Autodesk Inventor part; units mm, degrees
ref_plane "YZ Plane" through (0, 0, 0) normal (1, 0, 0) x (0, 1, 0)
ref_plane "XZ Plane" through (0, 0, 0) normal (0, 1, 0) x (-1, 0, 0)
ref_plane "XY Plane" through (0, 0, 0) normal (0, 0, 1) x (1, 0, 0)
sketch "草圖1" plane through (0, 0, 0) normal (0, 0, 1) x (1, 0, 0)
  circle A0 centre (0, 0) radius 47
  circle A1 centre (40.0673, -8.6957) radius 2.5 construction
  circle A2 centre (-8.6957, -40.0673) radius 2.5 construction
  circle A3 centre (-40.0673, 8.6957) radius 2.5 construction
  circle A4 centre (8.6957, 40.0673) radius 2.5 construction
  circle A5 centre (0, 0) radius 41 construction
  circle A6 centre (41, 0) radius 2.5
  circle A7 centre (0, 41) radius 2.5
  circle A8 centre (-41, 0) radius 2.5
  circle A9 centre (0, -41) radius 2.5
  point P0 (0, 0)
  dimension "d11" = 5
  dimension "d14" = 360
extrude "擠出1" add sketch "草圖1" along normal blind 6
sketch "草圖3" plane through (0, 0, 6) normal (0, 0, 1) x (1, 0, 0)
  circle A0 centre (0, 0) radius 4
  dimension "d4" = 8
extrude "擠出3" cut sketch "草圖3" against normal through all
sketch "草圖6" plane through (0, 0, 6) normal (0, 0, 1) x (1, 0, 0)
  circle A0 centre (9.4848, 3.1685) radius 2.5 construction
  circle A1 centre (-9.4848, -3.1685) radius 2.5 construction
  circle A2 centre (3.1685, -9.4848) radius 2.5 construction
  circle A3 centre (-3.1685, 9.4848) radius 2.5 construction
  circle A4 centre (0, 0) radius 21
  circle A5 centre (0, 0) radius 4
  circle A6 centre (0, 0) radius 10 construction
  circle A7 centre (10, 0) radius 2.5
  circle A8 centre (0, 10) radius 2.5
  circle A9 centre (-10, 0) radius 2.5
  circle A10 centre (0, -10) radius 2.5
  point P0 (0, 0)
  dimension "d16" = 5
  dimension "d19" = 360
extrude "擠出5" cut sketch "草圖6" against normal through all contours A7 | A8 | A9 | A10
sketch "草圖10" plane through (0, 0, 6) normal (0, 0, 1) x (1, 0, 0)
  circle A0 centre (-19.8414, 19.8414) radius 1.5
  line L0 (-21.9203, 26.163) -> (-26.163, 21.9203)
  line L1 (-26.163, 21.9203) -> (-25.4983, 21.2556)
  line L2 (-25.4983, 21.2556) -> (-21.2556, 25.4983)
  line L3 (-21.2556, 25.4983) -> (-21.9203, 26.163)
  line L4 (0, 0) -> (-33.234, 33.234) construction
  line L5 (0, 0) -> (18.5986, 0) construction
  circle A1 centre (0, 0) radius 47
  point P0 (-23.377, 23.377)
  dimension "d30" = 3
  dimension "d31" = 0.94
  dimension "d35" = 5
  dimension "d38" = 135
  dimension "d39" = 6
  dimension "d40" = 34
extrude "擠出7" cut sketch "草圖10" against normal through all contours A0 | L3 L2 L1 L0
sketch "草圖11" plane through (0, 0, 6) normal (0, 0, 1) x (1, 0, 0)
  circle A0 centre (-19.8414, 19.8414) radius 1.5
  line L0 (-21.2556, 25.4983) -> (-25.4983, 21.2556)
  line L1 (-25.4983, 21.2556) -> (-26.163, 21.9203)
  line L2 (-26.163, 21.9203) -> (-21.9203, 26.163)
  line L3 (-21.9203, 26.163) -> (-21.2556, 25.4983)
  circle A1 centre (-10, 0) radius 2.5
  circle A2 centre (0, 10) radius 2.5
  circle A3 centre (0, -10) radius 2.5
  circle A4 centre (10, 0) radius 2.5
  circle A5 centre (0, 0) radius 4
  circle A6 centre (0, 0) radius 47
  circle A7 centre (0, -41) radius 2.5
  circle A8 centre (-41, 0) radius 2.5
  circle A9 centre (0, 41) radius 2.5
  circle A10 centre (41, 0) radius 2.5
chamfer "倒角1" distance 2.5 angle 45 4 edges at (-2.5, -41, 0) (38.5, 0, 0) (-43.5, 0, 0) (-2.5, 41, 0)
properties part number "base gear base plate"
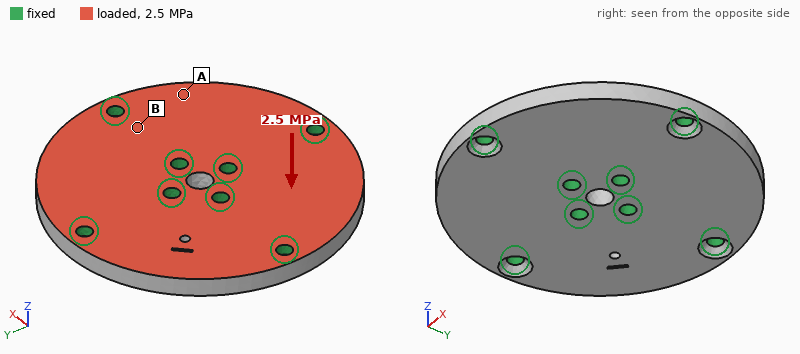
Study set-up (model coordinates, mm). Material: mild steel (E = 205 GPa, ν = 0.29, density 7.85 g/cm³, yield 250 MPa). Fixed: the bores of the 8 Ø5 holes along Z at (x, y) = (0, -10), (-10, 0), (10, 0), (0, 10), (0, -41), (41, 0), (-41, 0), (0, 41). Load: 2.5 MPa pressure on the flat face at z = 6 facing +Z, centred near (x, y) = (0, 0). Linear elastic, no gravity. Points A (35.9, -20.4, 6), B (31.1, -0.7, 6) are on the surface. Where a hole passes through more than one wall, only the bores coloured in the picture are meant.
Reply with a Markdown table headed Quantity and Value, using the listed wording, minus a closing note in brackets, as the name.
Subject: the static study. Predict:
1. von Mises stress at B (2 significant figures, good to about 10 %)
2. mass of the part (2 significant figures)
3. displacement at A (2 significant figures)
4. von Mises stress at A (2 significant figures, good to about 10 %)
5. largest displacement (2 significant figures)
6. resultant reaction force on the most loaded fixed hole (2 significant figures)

| Quantity | Value |
|---|---|
| von Mises stress at B | 74 MPa |
| mass of the part | 310 g |
| displacement at A | 24 µm |
| von Mises stress at A | 34 MPa |
| largest displacement | 38 µm |
| resultant reaction force on the most loaded fixed hole | 2.7 kN |
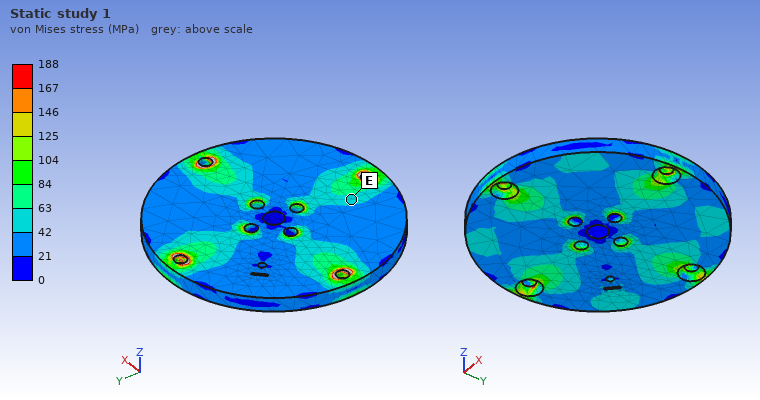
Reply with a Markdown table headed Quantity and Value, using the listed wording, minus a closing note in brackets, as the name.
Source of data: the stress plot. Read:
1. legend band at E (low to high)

| Quantity | Value |
|---|---|
| legend band at E | 42 to 63 MPa |
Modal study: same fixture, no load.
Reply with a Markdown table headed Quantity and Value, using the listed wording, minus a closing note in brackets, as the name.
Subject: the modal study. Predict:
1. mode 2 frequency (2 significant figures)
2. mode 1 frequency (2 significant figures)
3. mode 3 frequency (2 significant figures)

| Quantity | Value |
|---|---|
| mode 2 frequency | 7400 Hz |
| mode 1 frequency | 6600 Hz |
| mode 3 frequency | 7400 Hz |
